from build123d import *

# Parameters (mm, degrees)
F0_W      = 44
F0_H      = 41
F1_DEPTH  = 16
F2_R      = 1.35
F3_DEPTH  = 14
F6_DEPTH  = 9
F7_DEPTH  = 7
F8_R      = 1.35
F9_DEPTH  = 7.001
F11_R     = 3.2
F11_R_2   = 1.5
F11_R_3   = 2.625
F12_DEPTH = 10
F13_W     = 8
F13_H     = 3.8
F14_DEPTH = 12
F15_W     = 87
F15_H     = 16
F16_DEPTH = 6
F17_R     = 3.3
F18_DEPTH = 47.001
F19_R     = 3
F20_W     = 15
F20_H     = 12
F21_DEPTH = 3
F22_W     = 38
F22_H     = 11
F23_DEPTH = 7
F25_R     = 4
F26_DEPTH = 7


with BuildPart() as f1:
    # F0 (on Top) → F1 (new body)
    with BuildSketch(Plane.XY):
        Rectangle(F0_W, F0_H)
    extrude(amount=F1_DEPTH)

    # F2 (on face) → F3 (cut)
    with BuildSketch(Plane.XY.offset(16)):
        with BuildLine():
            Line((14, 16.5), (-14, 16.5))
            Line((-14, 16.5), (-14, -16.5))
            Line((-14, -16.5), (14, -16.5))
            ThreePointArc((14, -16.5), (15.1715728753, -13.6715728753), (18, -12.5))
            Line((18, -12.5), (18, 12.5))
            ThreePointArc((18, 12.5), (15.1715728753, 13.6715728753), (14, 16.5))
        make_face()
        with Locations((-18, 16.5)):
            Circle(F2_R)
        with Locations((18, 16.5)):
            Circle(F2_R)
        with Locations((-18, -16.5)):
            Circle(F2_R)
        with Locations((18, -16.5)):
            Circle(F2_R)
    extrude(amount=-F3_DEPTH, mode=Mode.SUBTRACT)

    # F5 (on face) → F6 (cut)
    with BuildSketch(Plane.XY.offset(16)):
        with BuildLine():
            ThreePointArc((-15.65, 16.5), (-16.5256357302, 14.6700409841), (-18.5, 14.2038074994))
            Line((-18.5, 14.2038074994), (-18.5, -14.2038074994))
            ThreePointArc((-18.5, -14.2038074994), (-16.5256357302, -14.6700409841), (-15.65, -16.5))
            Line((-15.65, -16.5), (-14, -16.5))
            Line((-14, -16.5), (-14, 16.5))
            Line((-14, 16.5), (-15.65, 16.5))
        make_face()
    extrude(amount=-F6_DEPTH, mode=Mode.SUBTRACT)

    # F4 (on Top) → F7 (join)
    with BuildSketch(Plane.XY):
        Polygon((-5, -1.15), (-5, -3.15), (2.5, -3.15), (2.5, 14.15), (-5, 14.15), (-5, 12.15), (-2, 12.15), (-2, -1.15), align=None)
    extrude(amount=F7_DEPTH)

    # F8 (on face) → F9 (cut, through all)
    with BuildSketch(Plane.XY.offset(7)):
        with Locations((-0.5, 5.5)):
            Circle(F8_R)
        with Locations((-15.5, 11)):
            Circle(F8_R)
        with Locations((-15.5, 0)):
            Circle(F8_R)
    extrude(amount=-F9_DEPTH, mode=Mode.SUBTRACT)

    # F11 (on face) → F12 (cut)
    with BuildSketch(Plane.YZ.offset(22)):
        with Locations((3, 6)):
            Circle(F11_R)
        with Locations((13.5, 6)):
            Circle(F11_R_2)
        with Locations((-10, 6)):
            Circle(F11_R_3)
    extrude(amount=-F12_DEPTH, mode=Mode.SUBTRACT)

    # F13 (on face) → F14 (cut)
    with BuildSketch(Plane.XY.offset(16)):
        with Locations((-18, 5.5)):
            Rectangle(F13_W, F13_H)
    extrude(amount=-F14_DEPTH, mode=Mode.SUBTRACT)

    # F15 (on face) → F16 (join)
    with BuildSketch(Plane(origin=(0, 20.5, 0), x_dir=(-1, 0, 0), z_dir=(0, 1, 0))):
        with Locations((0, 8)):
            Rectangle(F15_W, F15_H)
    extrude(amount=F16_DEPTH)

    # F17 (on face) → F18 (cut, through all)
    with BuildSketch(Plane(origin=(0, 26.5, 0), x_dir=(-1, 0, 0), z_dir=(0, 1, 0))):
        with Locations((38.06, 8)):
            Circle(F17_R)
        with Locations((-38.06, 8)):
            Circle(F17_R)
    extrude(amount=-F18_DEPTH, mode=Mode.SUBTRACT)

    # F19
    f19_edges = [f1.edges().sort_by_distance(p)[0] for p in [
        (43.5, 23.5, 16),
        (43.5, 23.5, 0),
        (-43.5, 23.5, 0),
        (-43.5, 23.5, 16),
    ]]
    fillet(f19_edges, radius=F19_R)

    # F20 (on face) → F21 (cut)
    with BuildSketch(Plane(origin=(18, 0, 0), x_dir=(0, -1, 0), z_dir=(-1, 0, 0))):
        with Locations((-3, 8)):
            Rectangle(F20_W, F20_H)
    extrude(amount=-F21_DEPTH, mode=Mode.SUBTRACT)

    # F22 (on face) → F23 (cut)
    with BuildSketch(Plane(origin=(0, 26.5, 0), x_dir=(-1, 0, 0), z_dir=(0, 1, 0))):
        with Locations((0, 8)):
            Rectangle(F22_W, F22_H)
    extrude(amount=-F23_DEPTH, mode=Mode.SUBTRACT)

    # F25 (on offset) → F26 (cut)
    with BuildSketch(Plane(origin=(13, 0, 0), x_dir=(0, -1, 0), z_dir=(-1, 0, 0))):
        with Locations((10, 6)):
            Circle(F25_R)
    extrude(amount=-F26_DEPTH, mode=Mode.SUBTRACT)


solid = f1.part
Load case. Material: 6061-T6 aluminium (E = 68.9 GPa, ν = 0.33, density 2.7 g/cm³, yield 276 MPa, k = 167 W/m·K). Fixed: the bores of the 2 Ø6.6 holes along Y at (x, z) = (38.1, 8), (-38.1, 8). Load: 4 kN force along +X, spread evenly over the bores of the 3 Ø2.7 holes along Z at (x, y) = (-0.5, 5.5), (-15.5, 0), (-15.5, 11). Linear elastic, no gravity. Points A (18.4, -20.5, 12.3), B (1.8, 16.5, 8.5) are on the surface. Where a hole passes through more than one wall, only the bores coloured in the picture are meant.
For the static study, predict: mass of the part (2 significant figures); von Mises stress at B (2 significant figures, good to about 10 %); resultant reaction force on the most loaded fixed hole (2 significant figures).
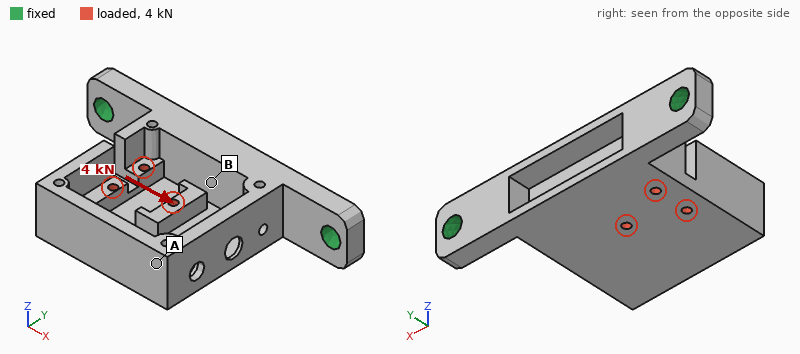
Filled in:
46 g
40 MPa
2.4 kN
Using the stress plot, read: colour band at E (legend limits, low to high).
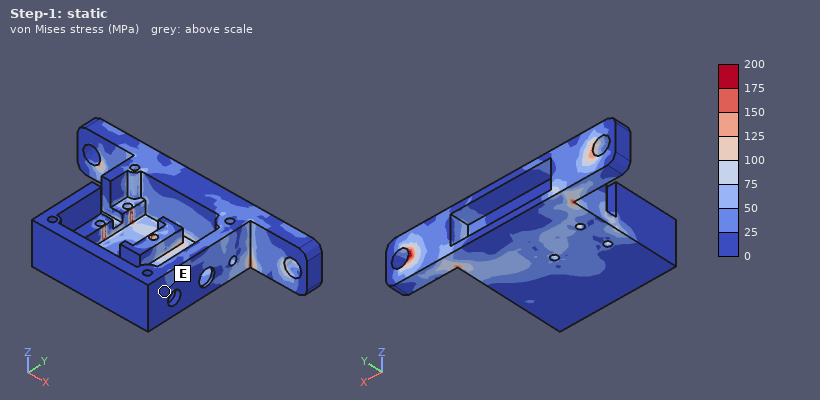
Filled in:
0 to 25 MPa
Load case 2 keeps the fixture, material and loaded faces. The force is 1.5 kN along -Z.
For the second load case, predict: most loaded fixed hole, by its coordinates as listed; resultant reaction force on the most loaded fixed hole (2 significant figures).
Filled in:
(-38.1, 8)
980 N
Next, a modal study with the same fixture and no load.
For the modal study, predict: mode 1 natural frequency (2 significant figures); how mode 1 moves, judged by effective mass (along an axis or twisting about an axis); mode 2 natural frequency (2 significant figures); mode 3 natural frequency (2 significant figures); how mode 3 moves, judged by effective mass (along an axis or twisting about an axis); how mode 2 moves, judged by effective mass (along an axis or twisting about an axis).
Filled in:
1400 Hz
along Z
3100 Hz
4900 Hz
along Y
along X
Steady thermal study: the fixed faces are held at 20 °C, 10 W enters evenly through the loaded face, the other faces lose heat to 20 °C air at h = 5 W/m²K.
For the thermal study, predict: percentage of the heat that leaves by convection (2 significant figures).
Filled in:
5.1 %
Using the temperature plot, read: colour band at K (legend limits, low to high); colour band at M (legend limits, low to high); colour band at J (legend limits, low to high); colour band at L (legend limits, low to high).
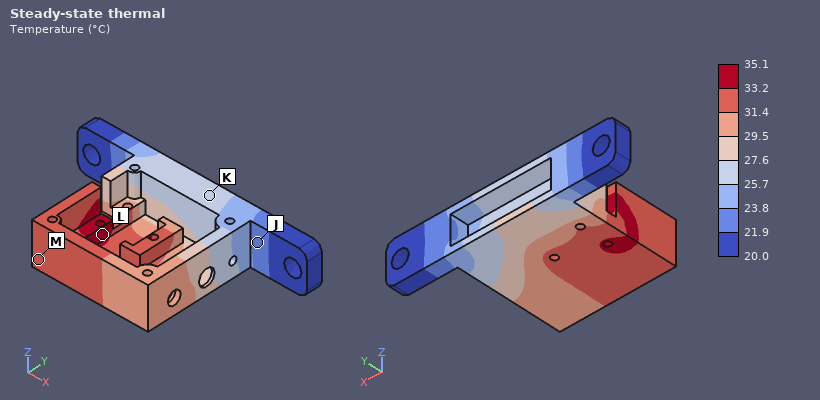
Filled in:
25.7 to 27.6 °C
31.4 to 33.2 °C
21.9 to 23.8 °C
33.2 to 35.1 °C
